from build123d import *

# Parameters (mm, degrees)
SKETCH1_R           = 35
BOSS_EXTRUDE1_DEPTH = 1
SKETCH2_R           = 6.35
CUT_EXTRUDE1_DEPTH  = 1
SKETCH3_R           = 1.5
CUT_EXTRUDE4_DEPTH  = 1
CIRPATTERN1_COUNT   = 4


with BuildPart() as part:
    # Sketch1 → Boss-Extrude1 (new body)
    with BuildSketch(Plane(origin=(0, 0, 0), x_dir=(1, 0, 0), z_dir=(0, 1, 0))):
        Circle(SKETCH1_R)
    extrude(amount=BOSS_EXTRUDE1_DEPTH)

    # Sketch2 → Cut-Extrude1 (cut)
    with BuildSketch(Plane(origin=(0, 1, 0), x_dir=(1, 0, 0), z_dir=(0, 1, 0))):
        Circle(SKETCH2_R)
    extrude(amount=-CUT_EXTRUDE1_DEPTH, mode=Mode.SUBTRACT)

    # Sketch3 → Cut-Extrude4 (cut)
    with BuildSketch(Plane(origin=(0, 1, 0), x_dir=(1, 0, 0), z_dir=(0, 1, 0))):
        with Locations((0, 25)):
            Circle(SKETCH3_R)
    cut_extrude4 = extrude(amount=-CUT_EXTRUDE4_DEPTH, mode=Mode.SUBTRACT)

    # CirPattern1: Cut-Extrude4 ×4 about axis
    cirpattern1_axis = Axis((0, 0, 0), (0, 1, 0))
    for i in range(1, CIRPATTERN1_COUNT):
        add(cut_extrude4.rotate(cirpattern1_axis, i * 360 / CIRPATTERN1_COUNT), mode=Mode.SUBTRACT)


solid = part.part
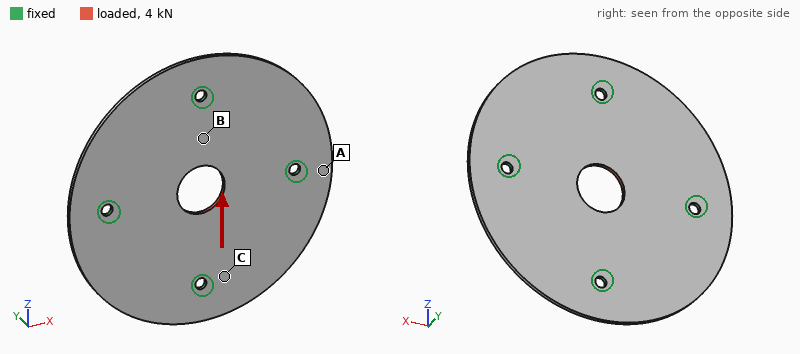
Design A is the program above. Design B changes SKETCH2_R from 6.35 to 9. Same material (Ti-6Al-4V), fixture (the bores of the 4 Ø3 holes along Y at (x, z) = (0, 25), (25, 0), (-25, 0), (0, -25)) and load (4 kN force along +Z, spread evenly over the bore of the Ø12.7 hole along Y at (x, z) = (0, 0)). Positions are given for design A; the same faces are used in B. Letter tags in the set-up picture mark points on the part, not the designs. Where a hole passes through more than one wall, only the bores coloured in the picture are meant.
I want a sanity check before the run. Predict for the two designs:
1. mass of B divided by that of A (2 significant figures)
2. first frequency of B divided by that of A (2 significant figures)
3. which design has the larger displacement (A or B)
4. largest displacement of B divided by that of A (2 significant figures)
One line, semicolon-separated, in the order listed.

0.97; 1.00; A; 0.85
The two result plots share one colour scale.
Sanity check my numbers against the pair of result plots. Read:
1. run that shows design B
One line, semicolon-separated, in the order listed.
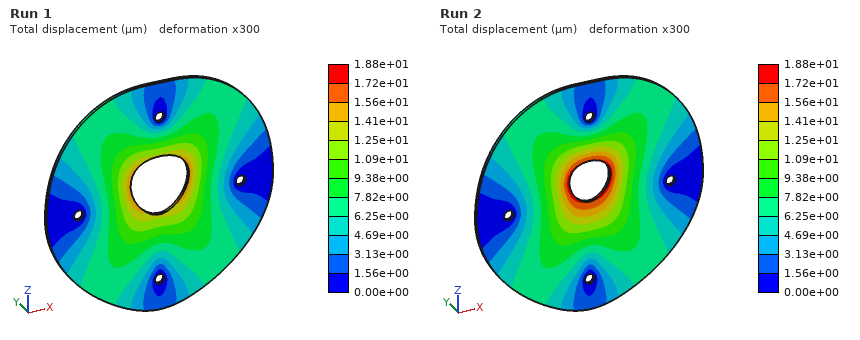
Run 1
